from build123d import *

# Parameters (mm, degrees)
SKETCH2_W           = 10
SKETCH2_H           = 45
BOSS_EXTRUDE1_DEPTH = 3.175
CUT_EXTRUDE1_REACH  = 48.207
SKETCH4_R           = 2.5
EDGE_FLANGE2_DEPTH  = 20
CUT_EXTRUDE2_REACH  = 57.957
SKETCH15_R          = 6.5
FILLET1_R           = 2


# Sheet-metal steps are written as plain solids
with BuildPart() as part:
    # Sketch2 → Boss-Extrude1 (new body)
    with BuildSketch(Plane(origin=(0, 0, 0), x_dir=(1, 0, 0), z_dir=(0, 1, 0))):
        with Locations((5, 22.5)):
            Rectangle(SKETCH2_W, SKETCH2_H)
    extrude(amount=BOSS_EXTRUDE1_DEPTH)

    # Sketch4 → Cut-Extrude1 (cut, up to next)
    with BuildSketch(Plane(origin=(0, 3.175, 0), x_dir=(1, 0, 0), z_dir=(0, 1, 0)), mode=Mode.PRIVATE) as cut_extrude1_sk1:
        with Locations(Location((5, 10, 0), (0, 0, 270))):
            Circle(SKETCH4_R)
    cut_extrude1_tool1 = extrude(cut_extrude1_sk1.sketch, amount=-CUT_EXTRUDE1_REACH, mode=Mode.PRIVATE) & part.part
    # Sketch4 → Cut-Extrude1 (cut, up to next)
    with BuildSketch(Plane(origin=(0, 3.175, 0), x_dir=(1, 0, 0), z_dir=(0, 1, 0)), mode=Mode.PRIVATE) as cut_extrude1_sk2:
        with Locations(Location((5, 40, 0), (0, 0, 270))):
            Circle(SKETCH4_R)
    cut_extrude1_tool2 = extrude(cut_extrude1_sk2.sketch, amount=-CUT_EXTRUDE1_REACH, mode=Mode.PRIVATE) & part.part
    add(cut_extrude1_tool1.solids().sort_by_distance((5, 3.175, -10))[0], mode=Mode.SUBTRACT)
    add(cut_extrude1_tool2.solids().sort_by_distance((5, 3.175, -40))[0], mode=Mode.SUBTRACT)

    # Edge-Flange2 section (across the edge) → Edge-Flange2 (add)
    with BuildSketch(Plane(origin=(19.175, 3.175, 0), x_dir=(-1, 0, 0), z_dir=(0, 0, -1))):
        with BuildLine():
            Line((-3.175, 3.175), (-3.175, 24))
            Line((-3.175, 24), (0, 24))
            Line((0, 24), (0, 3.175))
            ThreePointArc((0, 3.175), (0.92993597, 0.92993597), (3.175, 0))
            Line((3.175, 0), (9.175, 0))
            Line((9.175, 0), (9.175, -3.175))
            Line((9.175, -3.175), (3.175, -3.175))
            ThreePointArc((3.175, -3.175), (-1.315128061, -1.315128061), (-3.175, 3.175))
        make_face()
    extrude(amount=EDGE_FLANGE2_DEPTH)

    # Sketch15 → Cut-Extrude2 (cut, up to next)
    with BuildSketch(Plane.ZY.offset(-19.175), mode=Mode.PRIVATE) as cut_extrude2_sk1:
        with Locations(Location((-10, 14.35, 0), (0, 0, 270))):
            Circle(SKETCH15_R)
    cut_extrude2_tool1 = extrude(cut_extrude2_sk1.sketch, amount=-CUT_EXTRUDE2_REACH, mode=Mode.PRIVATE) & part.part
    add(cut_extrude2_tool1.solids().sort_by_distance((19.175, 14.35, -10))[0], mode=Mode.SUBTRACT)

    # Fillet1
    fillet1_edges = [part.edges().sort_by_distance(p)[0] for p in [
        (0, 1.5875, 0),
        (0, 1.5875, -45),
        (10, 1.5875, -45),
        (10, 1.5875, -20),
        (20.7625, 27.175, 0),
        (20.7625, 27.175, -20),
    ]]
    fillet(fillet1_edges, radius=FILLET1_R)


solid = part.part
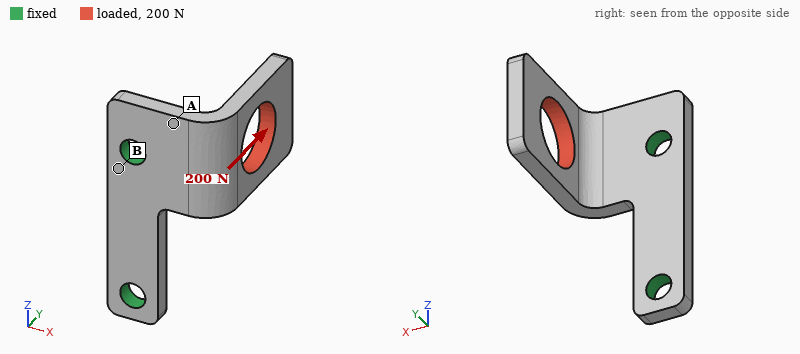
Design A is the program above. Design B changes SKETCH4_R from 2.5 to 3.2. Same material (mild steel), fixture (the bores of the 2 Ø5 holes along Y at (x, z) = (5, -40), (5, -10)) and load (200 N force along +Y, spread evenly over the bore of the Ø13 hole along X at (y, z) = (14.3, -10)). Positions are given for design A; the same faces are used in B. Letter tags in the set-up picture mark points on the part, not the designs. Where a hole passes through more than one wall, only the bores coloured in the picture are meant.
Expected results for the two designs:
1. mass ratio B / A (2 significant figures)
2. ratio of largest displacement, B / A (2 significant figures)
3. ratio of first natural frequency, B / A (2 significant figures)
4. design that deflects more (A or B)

0.97
0.88
1.0
A
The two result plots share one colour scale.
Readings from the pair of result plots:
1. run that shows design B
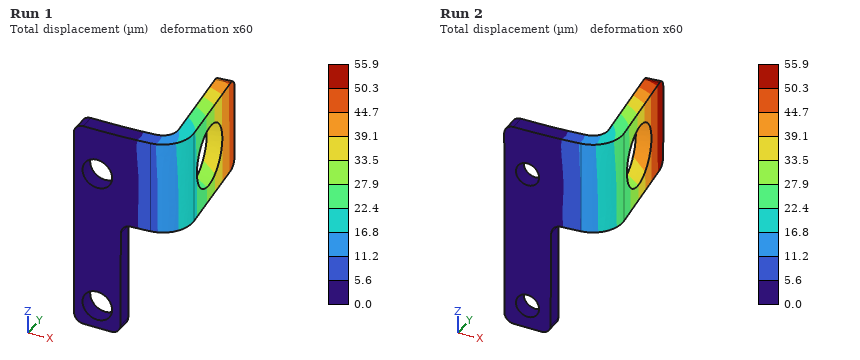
Run 1
